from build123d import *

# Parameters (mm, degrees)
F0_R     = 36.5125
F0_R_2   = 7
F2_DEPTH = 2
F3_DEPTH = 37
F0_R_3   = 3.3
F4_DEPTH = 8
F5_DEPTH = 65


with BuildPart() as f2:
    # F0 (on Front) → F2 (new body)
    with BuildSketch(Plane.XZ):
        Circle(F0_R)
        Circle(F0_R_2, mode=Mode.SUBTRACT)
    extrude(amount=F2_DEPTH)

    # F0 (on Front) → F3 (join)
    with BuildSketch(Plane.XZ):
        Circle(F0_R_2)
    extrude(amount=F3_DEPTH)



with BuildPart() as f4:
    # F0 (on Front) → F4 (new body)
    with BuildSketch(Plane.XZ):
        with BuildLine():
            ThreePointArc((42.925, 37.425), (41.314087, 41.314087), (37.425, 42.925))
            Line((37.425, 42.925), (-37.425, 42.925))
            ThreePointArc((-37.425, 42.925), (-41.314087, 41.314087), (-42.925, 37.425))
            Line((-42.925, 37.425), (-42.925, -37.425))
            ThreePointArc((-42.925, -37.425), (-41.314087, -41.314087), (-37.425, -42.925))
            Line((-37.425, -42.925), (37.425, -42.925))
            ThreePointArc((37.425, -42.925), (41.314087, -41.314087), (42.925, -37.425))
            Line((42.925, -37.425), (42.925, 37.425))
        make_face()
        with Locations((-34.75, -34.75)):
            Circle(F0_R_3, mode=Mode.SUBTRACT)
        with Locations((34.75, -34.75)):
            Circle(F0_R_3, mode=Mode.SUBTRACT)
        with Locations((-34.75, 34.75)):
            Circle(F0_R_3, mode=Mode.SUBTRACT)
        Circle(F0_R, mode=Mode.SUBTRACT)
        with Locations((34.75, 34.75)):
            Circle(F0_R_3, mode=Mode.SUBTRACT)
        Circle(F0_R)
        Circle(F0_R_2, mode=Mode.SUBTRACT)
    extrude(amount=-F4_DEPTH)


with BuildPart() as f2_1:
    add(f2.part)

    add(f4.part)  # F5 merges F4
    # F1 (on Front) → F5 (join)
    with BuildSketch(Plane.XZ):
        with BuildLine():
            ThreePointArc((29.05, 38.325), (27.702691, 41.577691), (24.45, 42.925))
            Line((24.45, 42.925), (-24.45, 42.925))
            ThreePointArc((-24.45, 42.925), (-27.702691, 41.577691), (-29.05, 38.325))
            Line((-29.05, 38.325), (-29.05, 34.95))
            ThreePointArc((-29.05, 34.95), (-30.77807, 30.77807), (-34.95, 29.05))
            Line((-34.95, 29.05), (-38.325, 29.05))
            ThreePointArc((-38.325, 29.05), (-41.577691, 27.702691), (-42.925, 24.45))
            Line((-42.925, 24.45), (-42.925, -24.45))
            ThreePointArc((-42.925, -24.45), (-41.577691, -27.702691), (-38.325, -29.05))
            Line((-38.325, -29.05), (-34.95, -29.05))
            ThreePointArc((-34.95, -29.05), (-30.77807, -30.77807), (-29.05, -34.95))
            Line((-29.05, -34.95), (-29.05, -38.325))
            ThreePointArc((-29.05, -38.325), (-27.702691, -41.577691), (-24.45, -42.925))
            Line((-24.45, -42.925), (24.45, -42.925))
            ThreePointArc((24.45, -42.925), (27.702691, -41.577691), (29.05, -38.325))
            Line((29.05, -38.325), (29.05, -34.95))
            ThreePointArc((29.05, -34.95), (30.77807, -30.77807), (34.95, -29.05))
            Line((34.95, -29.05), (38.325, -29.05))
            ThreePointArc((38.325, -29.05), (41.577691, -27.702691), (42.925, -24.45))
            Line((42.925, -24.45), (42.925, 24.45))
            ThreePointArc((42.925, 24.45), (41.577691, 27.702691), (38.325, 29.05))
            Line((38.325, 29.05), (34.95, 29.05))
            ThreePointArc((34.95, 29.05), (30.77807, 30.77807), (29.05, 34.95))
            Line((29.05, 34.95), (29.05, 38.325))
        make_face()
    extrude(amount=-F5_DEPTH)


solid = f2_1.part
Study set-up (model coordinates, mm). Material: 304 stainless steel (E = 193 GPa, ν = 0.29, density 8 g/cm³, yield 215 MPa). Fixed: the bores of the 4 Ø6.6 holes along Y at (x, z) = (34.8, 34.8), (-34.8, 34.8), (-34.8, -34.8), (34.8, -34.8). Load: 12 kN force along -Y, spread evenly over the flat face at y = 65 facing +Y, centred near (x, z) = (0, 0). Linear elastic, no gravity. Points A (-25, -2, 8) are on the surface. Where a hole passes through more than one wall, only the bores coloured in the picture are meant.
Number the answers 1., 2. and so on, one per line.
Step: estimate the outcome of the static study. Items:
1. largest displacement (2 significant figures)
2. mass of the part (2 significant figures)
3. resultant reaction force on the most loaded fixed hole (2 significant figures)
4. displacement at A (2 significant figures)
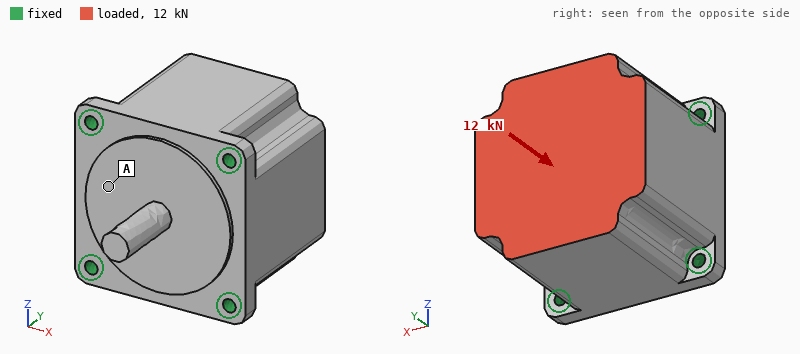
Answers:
1. 3.0 µm
2. 3.6 kg
3. 3.2 kN
4. 2.6 µm
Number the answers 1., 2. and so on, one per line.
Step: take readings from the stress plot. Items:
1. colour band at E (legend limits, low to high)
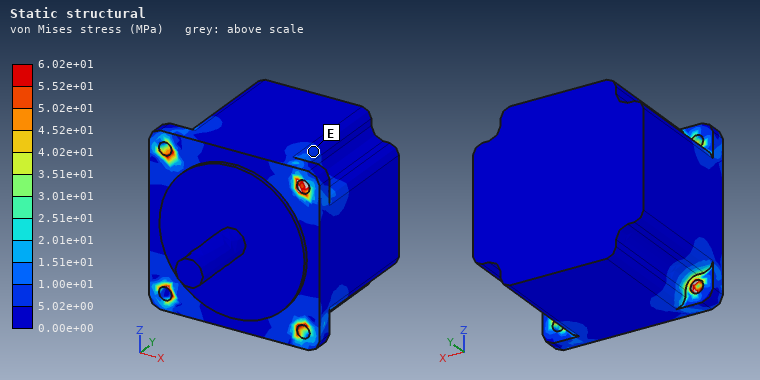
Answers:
1. 5.02e+00 to 1.00e+01 MPa
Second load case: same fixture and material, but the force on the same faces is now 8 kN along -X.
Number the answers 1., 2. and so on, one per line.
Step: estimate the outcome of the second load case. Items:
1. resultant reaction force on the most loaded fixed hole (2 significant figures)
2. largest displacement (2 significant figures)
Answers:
1. 4.3 kN
2. 8.8 µm
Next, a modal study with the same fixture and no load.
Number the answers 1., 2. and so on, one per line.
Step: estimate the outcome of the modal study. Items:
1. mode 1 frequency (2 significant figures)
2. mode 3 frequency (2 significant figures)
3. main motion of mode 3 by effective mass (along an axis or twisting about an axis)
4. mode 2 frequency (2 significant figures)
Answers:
1. 4400 Hz
2. 5700 Hz
3. along Y
4. 4400 Hz
